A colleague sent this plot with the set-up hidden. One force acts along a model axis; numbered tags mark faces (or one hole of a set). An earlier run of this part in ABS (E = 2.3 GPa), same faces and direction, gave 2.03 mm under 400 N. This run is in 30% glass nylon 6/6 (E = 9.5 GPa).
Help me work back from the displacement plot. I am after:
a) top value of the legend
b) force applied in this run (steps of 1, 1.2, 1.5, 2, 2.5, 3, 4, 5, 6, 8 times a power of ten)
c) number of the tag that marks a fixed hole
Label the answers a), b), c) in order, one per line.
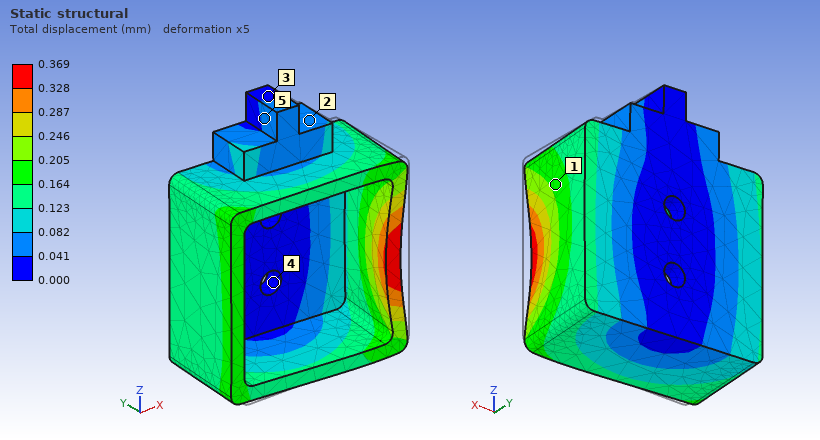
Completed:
a) 0.369 mm
b) 300 N
c) 4
